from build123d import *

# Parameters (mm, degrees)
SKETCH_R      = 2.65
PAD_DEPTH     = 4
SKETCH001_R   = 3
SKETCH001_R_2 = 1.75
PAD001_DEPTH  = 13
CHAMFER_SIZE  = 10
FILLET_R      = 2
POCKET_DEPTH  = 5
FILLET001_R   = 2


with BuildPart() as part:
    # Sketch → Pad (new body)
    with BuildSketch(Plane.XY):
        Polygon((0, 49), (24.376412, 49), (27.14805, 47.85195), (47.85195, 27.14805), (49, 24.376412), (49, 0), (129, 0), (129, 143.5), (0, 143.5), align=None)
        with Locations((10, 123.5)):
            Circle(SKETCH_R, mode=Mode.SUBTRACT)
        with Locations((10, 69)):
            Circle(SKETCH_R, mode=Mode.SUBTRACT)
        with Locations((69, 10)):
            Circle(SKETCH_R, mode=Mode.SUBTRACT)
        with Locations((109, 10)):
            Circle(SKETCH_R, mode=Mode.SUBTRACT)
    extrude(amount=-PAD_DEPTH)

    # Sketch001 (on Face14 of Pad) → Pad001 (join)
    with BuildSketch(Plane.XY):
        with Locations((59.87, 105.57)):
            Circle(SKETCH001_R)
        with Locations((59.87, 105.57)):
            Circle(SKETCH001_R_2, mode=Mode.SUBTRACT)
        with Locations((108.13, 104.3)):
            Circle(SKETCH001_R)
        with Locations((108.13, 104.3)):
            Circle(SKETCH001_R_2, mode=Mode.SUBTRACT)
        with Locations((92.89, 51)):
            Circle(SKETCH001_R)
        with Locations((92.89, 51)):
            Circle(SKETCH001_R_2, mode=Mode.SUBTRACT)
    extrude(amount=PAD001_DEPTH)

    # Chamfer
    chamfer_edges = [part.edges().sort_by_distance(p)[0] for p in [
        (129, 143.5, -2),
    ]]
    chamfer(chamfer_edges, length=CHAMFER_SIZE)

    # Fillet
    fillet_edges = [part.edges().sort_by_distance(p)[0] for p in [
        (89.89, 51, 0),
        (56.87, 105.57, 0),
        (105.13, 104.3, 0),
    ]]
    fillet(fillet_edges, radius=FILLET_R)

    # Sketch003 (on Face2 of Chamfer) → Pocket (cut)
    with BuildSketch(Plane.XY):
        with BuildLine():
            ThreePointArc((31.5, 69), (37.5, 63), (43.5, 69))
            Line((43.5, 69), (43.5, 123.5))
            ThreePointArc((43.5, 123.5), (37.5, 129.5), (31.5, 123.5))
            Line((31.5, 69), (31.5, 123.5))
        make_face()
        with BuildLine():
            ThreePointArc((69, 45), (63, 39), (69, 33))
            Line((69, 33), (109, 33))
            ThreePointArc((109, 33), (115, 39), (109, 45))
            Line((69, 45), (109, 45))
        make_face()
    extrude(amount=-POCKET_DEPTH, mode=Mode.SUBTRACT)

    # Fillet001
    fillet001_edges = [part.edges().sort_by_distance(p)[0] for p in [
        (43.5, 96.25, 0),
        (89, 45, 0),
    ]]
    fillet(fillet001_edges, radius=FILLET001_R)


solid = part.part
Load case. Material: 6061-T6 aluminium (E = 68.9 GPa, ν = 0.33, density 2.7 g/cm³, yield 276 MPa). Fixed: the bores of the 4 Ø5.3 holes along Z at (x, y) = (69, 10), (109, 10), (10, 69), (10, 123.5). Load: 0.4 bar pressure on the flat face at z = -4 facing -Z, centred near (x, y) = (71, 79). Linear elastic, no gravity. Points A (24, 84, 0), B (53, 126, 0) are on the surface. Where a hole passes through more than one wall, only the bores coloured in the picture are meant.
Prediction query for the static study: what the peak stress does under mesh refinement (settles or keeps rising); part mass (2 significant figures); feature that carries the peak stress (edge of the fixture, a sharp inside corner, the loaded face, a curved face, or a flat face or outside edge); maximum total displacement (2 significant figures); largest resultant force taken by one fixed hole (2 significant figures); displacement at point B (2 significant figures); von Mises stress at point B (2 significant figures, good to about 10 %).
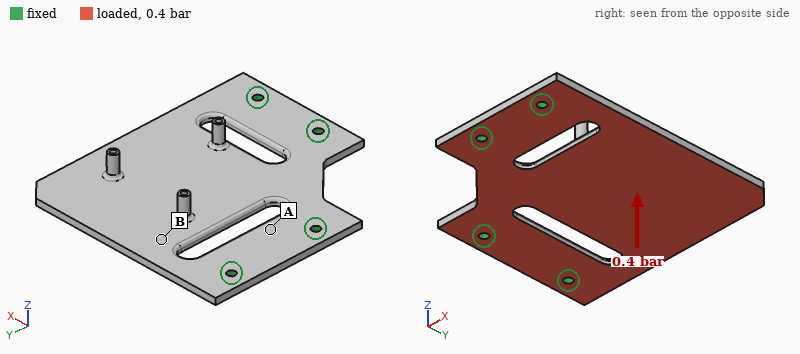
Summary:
keeps rising
160 g
edge of the fixture
1.5 mm
240 N
0.41 mm
21 MPa
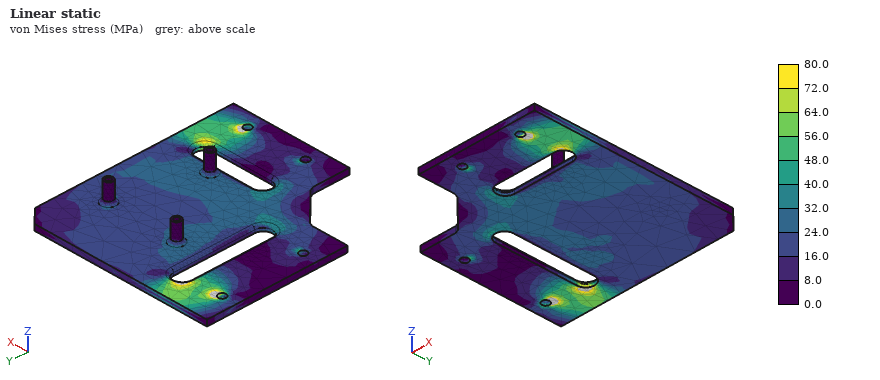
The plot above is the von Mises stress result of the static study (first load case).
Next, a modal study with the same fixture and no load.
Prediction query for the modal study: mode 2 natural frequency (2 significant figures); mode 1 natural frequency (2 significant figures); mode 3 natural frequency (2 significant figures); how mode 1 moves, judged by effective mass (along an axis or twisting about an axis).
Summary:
1200 Hz
340 Hz
1400 Hz
along Z
